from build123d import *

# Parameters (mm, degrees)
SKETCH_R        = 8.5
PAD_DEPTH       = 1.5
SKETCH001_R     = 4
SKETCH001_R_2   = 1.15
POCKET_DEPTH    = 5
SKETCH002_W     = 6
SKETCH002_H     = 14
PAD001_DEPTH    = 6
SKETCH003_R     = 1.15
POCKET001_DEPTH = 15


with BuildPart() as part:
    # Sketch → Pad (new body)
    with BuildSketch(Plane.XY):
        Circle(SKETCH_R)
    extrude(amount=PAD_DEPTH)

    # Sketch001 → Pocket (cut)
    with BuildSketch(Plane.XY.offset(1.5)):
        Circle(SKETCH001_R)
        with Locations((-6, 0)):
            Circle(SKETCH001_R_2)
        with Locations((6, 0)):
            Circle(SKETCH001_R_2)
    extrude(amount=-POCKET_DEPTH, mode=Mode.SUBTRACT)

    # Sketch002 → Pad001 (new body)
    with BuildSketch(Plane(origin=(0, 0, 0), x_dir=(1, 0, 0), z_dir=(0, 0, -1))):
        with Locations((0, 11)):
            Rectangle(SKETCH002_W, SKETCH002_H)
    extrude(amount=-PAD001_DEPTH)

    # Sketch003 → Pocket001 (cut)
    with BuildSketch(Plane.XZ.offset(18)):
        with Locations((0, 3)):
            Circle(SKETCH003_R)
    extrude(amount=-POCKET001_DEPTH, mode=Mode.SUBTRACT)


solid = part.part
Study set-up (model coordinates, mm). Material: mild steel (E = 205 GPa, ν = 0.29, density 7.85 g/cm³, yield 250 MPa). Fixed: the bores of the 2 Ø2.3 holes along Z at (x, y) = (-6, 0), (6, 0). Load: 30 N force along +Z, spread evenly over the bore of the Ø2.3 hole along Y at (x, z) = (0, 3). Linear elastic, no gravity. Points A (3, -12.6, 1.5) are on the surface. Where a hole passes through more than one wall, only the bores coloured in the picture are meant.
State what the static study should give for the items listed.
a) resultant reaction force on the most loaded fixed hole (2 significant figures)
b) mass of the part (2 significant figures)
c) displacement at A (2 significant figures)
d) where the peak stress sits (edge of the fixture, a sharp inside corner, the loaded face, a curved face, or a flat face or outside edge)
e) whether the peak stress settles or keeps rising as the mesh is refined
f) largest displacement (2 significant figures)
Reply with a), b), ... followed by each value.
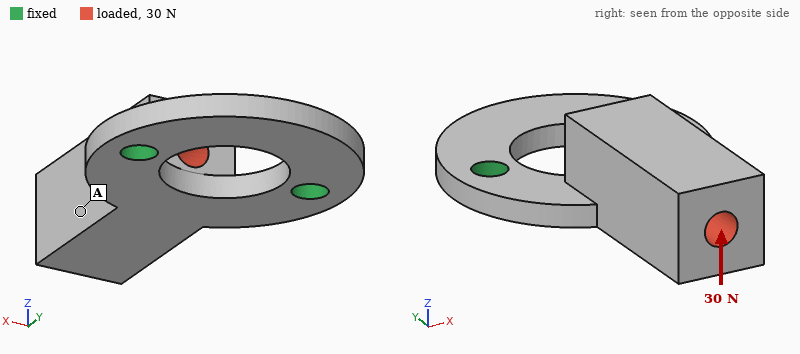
a) 15 N
b) 5.2 g
c) 24 µm
d) edge of the fixture
e) keeps rising
f) 39 µm
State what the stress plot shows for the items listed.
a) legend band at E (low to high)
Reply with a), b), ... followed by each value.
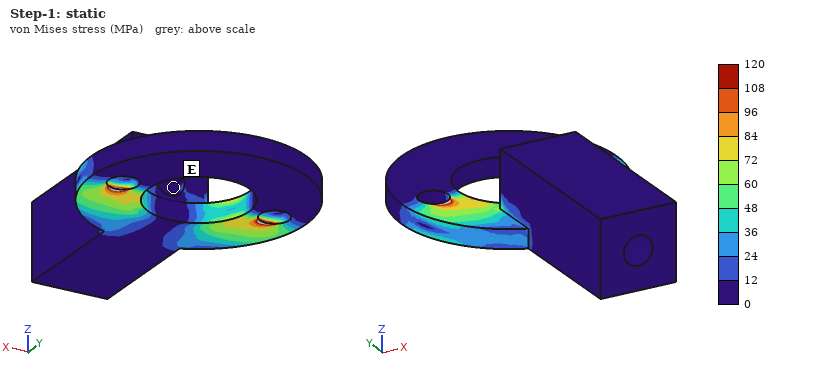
a) 0 to 12 MPa
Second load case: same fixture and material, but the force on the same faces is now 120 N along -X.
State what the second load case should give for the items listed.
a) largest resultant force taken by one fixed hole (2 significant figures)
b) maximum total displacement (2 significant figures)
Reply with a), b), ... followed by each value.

a) 120 N
b) 6.3 µm
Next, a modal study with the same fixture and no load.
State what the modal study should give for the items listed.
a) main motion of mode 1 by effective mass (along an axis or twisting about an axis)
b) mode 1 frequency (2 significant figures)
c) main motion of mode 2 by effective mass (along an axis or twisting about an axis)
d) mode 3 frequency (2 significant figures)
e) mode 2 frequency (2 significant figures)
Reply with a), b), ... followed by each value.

a) along Z
b) 2800 Hz
c) along X
d) 18 kHz
e) 15 kHz
